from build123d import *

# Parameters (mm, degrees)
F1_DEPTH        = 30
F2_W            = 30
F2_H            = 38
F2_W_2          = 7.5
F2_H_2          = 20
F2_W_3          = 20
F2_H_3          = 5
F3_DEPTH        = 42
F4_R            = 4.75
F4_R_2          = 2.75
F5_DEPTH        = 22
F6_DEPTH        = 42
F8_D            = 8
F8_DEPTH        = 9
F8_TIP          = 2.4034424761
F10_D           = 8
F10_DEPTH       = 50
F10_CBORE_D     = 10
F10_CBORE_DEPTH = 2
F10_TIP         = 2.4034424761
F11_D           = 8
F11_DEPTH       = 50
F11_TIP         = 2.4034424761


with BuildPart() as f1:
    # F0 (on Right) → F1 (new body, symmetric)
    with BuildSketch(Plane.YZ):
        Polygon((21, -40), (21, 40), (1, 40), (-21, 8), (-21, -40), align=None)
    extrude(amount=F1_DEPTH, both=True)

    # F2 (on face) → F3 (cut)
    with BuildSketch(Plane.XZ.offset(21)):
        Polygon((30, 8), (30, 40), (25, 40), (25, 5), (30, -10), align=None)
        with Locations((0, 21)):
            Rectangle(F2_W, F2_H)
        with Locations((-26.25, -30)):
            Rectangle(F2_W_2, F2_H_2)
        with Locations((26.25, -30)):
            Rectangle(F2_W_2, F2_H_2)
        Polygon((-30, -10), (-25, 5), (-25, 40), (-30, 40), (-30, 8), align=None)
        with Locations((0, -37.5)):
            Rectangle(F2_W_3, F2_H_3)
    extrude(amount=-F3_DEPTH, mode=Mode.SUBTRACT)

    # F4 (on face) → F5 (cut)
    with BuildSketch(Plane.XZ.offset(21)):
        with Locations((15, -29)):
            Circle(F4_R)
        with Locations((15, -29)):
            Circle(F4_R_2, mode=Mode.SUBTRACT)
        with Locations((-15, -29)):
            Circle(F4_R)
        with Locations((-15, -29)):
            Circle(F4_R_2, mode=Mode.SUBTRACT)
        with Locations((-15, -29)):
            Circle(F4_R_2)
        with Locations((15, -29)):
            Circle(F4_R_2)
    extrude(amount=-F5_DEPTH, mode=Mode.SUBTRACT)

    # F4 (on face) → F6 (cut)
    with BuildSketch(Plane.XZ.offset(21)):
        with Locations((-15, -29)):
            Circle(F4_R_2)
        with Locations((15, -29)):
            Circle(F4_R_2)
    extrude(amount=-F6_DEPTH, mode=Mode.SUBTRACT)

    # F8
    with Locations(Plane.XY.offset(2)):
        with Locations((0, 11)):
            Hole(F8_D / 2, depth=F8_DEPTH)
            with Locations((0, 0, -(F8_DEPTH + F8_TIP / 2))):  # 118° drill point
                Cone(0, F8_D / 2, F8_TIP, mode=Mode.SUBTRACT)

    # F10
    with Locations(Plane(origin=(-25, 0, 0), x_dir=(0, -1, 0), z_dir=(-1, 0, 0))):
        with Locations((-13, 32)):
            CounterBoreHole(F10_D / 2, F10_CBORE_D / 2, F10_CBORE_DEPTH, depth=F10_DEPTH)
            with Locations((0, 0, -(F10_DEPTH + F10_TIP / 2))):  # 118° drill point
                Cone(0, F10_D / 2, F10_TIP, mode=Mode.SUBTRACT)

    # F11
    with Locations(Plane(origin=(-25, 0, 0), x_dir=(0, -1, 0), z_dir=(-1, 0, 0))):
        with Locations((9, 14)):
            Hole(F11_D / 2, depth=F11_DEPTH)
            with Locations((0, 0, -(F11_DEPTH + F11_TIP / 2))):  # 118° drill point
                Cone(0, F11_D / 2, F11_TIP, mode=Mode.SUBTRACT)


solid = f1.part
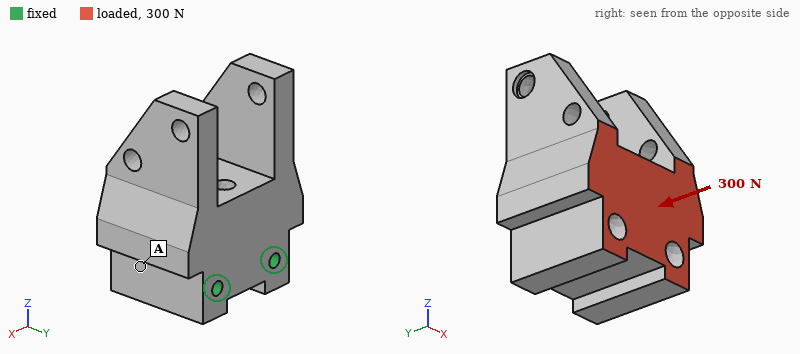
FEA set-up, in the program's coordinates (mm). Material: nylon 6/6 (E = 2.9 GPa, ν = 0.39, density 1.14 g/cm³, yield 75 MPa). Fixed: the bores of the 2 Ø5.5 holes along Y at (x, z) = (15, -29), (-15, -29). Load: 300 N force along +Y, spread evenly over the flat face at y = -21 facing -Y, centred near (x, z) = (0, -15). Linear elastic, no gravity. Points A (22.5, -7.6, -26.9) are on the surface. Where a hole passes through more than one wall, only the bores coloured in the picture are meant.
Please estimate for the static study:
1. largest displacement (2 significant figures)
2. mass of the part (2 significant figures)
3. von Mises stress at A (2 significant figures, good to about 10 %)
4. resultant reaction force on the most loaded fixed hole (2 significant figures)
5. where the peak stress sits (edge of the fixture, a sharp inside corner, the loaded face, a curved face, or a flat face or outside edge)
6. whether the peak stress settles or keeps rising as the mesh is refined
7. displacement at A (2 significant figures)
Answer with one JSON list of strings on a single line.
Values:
["36 µm", "120 g", "0.40 MPa", "150 N", "edge of the fixture", "keeps rising", "7.9 µm"]
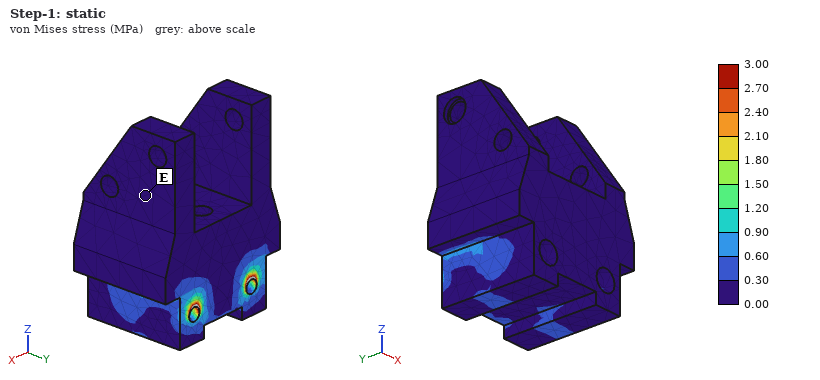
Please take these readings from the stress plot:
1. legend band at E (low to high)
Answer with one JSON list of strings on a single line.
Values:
["0.00 to 0.30 MPa"]
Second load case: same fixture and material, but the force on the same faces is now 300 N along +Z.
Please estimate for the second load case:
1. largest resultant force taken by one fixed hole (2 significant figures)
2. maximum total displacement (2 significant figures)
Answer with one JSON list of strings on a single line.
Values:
["150 N", "77 µm"]
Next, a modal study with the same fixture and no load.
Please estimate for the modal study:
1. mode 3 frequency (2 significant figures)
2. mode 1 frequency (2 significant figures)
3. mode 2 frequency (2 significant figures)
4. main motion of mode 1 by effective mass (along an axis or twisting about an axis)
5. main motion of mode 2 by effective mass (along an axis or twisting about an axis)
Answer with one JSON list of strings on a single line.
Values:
["1700 Hz", "1300 Hz", "1500 Hz", "along Y", "along X"]
